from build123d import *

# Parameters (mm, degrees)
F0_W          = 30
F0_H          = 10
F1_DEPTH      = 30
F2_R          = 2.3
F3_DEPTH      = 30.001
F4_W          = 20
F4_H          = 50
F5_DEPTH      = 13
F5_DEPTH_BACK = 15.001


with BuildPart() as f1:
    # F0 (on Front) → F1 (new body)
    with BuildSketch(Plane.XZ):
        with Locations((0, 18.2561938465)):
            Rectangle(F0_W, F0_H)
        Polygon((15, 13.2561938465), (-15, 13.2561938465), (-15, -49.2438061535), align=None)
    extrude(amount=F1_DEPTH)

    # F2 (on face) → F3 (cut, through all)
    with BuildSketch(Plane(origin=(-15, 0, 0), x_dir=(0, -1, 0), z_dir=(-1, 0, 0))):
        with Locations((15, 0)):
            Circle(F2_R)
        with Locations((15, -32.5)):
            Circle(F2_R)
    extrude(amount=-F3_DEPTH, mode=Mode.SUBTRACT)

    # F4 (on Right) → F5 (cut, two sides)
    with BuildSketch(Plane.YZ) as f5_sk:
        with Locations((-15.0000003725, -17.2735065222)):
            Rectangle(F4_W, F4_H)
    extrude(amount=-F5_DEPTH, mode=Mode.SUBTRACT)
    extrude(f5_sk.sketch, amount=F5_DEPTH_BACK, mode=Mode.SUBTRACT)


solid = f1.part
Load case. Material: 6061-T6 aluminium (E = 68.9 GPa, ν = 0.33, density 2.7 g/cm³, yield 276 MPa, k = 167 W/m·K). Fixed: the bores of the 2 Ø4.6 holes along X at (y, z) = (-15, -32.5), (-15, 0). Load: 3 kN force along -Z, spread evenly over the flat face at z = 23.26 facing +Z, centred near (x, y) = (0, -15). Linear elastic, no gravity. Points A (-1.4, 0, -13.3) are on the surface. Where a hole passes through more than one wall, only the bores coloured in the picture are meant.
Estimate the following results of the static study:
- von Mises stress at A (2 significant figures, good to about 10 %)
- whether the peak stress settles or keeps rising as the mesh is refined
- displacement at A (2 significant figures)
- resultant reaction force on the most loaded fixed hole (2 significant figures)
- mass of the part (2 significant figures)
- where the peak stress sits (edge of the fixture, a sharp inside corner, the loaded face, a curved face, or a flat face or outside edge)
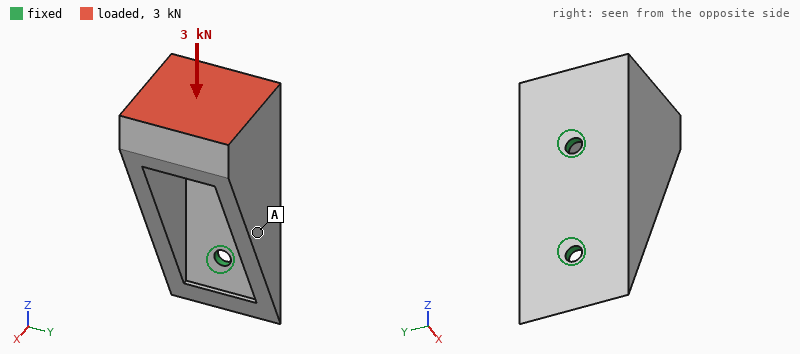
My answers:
32 MPa
keeps rising
0.064 mm
2.0 kN
64 g
edge of the fixture
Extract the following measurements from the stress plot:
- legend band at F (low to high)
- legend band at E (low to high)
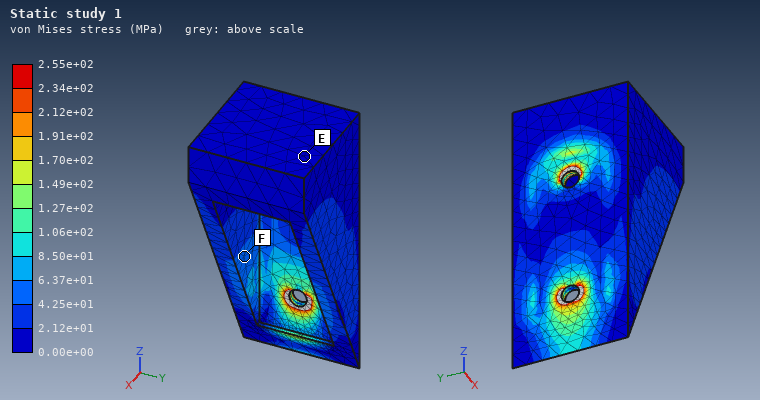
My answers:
4.25e+01 to 6.37e+01 MPa
0.00e+00 to 2.12e+01 MPa
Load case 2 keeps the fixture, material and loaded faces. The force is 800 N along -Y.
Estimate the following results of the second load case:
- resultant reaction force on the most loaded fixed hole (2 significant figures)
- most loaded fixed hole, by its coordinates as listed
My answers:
1.3 kN
(-15, 0)
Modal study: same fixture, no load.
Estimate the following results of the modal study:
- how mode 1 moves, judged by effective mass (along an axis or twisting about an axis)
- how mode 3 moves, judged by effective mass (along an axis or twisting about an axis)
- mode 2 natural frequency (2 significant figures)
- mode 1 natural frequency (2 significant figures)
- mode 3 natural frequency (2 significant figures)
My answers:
along Y
along X
2400 Hz
1200 Hz
5000 Hz
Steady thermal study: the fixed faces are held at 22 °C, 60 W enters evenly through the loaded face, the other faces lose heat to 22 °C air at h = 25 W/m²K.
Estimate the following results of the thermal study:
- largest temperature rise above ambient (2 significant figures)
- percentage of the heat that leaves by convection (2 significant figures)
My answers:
50 K
10 %
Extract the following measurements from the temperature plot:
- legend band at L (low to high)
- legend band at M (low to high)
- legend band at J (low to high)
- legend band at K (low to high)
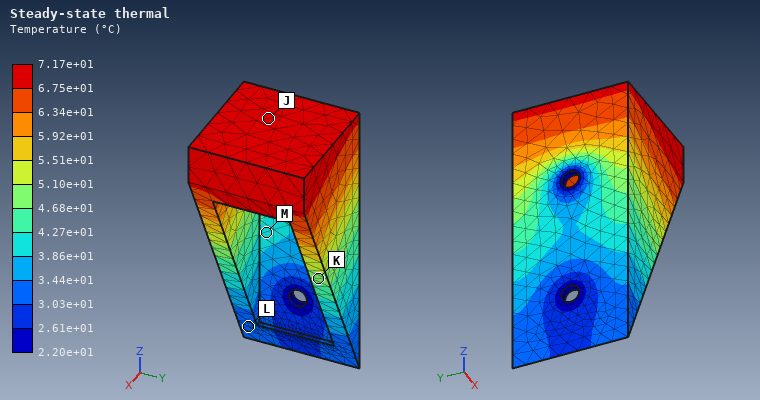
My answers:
3.03e+01 to 3.44e+01 °C
3.86e+01 to 4.27e+01 °C
6.75e+01 to 7.17e+01 °C
4.68e+01 to 5.10e+01 °C
